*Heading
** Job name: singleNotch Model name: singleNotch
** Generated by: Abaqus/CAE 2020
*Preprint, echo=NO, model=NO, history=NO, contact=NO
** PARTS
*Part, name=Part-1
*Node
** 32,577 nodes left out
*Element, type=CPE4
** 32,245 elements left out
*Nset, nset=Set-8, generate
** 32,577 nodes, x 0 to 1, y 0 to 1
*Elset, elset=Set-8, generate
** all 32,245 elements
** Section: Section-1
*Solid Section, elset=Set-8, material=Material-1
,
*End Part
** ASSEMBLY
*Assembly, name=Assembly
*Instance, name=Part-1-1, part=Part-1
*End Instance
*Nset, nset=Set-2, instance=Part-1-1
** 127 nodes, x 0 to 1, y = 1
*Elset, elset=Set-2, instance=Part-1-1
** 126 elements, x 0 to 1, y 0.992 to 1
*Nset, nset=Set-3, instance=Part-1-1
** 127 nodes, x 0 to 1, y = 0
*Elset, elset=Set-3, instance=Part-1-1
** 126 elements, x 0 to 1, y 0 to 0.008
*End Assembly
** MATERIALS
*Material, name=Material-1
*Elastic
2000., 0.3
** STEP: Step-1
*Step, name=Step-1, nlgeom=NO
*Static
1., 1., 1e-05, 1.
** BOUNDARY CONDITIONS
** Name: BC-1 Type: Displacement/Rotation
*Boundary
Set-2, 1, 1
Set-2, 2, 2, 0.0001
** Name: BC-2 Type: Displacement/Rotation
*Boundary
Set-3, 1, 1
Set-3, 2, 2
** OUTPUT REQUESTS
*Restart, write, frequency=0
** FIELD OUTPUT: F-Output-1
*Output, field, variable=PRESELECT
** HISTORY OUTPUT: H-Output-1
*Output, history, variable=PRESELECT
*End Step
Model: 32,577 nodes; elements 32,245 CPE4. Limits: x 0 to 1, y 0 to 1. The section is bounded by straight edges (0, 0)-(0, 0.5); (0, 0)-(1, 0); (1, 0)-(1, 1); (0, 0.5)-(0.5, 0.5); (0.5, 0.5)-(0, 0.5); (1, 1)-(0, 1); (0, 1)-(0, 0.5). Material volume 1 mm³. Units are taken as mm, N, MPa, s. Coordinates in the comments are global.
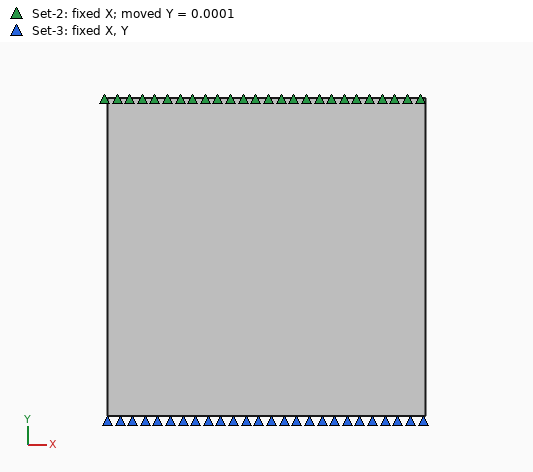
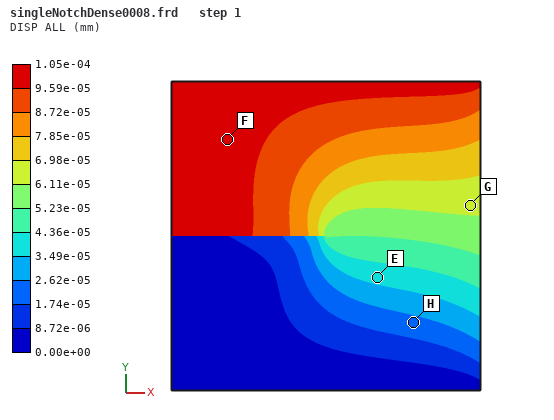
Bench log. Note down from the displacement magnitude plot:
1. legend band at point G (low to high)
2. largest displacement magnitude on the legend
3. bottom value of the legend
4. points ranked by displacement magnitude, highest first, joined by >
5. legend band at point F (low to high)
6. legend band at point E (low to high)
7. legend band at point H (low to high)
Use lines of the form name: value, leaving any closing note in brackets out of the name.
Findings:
legend band at point G: 6.11e-05 to 6.98e-05 mm
largest displacement magnitude on the legend: 1.05e-04 mm
bottom value of the legend: 0.00e+00 mm
points ranked by displacement magnitude, highest first, joined by >: F > G > E > H
legend band at point F: 9.59e-05 to 1.05e-04 mm
legend band at point E: 3.49e-05 to 4.36e-05 mm
legend band at point H: 1.74e-05 to 2.62e-05 mm
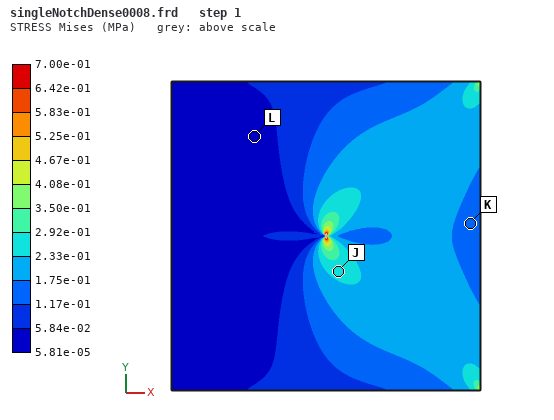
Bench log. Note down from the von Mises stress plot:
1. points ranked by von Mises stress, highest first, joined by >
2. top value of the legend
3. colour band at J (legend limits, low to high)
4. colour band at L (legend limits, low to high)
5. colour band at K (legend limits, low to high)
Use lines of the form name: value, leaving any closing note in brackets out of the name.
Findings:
points ranked by von Mises stress, highest first, joined by >: J > K > L
top value of the legend: 7.00e-01 MPa
colour band at J: 2.33e-01 to 2.92e-01 MPa
colour band at L: 5.81e-05 to 5.84e-02 MPa
colour band at K: 1.17e-01 to 1.75e-01 MPa
